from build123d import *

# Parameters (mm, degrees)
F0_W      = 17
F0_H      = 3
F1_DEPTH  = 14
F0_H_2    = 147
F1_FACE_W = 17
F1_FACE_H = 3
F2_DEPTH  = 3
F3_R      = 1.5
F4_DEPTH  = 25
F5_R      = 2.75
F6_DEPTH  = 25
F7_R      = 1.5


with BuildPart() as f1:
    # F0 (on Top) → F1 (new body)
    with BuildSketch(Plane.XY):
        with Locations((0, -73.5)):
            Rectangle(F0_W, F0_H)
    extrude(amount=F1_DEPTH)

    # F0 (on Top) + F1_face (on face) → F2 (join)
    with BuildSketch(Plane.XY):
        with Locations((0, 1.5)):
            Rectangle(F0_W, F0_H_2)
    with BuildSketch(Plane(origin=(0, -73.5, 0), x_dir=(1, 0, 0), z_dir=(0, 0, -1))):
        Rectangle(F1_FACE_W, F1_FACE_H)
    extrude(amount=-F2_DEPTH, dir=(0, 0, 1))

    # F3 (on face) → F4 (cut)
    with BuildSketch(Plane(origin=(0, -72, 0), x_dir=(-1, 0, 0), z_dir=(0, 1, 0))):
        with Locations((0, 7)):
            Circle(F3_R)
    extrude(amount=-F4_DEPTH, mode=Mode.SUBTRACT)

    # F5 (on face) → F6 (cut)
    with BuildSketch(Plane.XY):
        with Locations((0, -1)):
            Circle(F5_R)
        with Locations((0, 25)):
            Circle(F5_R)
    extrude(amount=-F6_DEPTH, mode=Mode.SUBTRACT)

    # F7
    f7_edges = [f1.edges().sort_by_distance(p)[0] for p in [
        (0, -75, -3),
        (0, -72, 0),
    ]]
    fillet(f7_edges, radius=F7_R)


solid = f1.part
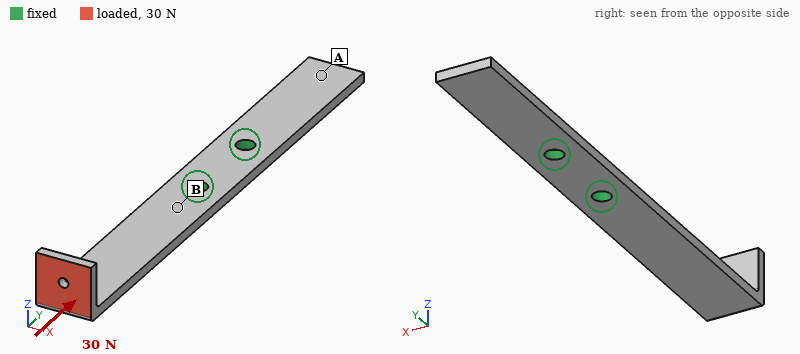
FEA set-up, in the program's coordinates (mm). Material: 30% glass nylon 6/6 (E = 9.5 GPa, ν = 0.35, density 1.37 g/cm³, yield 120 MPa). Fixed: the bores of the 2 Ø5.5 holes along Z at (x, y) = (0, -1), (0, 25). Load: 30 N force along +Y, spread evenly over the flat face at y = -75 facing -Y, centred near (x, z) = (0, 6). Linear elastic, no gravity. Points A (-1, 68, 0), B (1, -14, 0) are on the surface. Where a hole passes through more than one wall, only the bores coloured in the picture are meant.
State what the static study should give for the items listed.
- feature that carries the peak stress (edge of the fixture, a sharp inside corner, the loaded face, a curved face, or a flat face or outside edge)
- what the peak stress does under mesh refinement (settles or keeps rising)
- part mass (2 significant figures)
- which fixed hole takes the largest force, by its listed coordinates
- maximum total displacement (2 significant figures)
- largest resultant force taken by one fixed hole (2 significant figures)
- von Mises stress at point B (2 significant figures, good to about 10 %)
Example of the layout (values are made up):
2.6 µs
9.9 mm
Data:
edge of the fixture
keeps rising
11 g
(0, -1)
1.8 mm
28 N
9.3 MPa
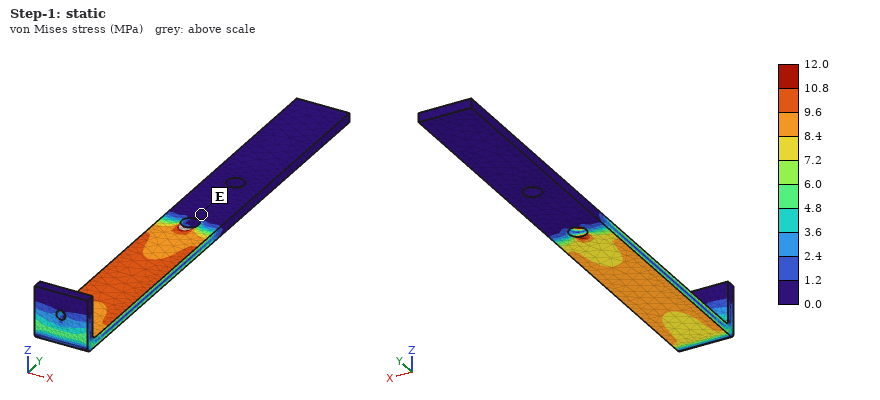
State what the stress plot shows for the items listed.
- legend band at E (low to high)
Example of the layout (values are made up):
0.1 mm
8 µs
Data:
0.0 to 1.2 MPa
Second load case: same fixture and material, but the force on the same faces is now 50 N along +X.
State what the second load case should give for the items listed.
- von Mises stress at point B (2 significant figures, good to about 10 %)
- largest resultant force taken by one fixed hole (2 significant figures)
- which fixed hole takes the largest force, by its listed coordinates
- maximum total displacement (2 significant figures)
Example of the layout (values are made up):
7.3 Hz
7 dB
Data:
17 MPa
120 N
(0, -1)
1.6 mm
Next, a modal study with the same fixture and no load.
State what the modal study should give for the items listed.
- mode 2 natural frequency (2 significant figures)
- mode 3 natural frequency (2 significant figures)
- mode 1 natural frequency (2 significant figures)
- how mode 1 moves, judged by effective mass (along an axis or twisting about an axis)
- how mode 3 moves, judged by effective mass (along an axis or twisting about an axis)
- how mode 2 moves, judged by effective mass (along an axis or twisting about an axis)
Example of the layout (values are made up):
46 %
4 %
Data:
550 Hz
800 Hz
190 Hz
along Z
along X
along Z
